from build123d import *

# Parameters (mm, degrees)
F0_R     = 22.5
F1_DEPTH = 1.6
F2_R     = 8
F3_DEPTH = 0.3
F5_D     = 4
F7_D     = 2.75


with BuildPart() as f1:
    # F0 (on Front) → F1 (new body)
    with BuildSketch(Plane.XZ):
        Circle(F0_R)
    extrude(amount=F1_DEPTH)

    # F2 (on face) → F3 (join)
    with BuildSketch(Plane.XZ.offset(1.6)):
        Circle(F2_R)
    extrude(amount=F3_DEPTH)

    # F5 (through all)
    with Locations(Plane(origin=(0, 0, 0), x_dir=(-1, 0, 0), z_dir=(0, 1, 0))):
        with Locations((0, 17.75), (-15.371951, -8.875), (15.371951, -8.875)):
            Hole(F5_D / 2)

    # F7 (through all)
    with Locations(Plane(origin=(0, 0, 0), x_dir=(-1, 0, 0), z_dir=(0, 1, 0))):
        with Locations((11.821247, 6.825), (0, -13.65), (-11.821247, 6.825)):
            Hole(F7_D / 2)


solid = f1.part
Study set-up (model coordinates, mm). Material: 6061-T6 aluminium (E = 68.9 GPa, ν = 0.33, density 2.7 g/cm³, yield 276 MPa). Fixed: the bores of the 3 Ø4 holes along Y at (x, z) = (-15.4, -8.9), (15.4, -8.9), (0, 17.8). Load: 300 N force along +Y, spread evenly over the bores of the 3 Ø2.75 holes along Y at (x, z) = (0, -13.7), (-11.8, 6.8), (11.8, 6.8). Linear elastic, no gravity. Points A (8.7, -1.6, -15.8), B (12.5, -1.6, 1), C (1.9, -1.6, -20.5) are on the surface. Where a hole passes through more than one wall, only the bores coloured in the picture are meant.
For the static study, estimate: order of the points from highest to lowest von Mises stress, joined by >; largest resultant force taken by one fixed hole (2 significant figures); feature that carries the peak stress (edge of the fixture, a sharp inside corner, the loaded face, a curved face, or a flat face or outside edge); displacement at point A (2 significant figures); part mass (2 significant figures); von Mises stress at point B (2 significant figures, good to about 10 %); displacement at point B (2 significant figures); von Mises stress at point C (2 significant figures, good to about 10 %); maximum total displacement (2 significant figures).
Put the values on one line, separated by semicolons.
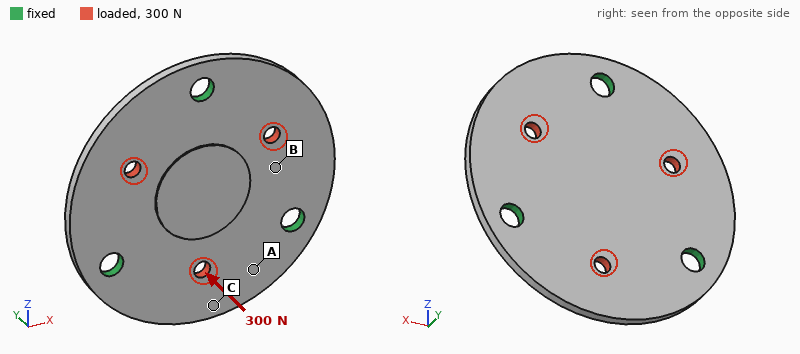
C > B > A; 100 N; the loaded face; 23 µm; 6.8 g; 18 MPa; 25 µm; 33 MPa; 57 µm
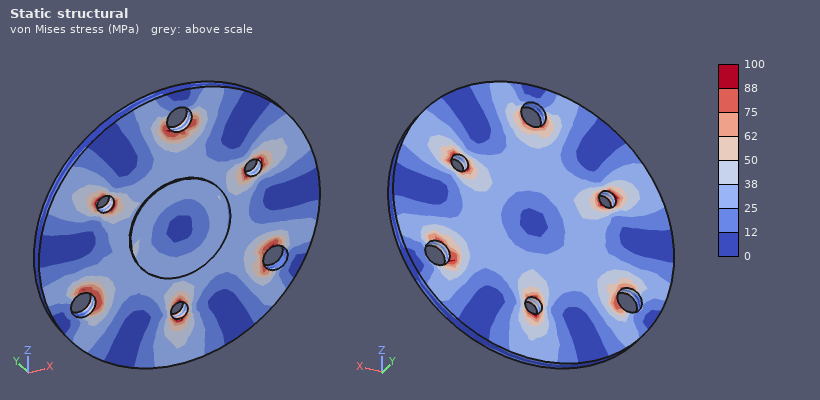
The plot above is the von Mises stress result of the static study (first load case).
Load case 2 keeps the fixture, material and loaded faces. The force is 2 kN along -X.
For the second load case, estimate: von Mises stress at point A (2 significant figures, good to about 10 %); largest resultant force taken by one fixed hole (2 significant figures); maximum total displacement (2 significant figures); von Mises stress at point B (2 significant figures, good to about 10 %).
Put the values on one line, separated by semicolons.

17 MPa; 710 N; 9.5 µm; 14 MPa
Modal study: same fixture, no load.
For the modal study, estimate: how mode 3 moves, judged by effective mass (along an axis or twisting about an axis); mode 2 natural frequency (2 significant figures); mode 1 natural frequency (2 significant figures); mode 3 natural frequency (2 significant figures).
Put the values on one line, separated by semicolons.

along Y; 6500 Hz; 6500 Hz; 7000 Hz
